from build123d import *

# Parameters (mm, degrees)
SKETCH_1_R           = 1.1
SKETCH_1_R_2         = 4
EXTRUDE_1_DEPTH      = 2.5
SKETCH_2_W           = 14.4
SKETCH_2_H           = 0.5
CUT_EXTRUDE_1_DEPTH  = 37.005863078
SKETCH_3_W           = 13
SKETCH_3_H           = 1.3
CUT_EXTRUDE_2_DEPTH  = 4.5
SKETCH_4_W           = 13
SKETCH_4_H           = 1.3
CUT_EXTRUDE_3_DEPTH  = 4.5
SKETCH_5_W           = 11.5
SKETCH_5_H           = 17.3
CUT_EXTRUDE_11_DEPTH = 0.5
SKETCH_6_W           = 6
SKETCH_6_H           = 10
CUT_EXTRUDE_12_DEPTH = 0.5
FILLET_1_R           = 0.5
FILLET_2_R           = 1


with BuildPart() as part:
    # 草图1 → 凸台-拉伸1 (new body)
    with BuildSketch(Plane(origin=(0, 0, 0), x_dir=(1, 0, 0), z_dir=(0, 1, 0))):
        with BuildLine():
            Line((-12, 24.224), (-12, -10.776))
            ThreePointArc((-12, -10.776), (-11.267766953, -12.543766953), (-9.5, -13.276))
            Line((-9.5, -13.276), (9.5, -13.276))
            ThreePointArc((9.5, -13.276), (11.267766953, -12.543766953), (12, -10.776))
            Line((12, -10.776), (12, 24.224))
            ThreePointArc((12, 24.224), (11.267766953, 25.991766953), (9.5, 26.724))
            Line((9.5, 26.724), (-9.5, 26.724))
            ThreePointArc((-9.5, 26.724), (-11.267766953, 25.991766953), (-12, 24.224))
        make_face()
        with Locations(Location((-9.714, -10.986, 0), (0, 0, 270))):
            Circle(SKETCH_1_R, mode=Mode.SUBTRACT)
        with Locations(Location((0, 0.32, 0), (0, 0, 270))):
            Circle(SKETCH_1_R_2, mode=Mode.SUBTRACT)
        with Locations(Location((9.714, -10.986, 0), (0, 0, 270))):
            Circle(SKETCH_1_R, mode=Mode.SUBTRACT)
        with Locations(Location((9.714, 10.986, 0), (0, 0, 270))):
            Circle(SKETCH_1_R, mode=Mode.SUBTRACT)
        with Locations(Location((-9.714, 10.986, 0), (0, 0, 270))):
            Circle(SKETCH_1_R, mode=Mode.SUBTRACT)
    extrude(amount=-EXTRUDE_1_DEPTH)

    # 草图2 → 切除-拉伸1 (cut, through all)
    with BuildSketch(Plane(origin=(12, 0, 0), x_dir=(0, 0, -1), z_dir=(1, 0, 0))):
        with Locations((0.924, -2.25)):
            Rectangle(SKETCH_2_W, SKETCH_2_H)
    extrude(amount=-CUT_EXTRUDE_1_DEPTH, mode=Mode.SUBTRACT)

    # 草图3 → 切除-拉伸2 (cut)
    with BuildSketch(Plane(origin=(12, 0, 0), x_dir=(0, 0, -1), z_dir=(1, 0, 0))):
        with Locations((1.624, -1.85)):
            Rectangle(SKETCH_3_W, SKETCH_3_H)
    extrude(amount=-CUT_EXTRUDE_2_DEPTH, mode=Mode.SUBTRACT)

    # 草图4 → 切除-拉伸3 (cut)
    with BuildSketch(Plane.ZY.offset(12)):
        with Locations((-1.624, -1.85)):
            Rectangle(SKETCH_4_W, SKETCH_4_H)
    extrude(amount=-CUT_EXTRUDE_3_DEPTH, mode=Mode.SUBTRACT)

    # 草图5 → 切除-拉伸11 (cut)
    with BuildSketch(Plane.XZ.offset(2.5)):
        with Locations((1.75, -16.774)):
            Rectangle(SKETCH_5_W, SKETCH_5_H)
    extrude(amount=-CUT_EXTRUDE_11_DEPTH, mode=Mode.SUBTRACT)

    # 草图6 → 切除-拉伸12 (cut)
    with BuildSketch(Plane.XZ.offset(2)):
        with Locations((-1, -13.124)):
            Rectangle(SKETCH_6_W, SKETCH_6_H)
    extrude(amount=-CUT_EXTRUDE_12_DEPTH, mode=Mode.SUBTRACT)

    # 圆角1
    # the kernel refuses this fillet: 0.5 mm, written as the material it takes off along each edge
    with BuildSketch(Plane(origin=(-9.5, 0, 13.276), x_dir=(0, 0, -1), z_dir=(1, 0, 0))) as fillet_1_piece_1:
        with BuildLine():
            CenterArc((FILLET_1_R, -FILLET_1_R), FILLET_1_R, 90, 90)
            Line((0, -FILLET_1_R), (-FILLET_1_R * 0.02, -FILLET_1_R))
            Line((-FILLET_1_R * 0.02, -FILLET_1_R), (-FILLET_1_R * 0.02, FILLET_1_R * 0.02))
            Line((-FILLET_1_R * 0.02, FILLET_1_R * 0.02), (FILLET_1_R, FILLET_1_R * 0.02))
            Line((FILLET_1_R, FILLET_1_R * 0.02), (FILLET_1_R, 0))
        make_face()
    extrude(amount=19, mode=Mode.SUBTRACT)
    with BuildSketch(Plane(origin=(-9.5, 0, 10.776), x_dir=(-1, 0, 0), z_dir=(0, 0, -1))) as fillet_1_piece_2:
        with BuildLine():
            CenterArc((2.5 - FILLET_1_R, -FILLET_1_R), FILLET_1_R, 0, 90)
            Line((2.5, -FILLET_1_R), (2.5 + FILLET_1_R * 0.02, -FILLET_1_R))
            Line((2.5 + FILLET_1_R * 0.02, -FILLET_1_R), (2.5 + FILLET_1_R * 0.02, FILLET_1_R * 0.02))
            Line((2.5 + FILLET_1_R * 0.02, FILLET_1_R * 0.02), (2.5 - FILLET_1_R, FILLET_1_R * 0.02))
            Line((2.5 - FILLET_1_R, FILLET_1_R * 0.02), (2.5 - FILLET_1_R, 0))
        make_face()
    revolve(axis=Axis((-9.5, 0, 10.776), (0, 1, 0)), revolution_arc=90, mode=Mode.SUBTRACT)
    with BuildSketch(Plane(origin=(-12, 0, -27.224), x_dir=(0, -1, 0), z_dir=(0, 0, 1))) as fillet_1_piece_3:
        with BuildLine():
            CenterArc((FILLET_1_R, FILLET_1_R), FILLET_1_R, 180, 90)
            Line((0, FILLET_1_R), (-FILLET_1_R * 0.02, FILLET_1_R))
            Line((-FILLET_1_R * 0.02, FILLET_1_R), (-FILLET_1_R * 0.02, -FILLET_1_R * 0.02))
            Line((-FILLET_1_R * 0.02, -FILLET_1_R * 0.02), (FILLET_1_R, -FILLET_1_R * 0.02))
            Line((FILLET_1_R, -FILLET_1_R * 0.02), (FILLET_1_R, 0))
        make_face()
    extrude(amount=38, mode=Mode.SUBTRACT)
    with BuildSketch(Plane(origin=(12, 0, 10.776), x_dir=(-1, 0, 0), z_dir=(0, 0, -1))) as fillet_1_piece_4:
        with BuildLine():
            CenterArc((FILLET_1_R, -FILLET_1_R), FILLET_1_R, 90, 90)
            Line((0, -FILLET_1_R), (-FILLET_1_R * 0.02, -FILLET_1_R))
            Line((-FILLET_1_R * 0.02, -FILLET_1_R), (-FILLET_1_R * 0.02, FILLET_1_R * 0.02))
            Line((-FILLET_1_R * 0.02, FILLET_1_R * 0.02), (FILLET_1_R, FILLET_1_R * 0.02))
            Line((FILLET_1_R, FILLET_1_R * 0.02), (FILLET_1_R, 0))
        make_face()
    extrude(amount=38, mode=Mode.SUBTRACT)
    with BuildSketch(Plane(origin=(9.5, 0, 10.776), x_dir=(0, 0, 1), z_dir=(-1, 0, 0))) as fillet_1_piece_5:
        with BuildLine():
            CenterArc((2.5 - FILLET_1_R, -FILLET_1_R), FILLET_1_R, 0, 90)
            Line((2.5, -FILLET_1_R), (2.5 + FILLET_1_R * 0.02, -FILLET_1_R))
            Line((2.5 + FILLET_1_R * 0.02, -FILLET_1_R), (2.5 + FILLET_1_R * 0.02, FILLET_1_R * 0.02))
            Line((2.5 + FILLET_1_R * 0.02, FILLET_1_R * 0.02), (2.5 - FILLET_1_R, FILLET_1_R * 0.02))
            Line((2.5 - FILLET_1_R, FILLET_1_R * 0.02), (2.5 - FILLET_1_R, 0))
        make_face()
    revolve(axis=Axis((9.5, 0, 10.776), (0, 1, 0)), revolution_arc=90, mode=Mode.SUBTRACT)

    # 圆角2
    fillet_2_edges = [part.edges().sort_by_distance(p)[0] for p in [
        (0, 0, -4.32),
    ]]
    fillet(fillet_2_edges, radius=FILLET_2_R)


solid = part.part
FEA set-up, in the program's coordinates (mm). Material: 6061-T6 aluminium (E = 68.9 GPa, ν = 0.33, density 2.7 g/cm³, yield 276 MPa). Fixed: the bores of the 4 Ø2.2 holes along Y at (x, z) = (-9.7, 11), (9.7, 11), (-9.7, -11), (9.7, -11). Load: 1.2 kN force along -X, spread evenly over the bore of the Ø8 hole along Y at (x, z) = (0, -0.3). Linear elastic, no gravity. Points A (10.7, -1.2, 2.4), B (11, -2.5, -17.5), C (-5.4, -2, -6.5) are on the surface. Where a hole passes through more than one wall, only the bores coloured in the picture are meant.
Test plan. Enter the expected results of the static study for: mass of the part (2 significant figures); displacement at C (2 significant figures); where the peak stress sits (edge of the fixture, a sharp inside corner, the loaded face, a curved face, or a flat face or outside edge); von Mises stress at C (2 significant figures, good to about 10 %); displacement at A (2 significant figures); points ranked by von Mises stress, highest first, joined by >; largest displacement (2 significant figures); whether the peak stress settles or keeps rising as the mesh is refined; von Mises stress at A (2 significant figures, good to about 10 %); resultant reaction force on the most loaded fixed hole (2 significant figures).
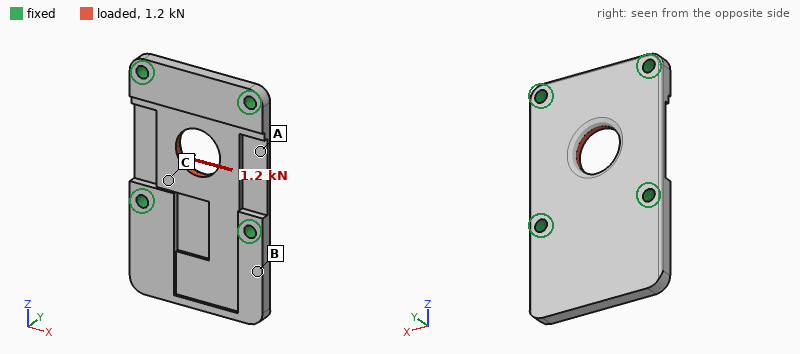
5.0 g
3.7 µm
edge of the fixture
37 MPa
5.7 µm
C > A > B
8.7 µm
keeps rising
16 MPa
360 N
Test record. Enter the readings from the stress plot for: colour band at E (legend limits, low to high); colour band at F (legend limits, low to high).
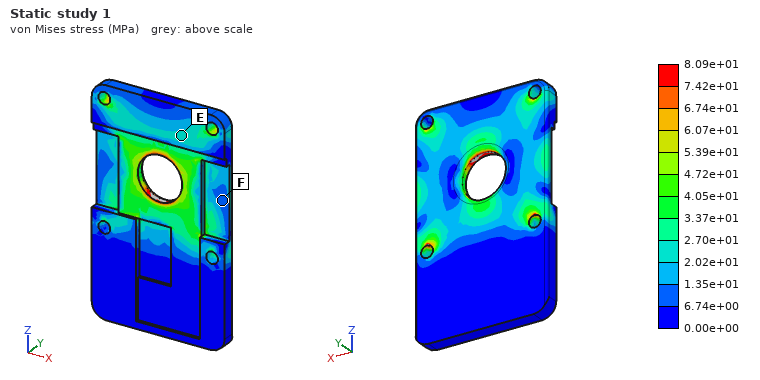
2.02e+01 to 2.70e+01 MPa
6.74e+00 to 1.35e+01 MPa
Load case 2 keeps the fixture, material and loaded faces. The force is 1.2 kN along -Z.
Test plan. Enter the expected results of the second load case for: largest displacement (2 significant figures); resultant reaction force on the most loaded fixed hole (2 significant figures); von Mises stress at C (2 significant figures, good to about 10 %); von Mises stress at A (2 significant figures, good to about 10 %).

6.2 µm
330 N
34 MPa
13 MPa
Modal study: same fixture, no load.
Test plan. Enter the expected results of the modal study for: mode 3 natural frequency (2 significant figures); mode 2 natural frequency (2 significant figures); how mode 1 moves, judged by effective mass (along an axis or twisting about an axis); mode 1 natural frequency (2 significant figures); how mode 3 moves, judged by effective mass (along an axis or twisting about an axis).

20 kHz
14 kHz
along Y
7000 Hz
along Y
